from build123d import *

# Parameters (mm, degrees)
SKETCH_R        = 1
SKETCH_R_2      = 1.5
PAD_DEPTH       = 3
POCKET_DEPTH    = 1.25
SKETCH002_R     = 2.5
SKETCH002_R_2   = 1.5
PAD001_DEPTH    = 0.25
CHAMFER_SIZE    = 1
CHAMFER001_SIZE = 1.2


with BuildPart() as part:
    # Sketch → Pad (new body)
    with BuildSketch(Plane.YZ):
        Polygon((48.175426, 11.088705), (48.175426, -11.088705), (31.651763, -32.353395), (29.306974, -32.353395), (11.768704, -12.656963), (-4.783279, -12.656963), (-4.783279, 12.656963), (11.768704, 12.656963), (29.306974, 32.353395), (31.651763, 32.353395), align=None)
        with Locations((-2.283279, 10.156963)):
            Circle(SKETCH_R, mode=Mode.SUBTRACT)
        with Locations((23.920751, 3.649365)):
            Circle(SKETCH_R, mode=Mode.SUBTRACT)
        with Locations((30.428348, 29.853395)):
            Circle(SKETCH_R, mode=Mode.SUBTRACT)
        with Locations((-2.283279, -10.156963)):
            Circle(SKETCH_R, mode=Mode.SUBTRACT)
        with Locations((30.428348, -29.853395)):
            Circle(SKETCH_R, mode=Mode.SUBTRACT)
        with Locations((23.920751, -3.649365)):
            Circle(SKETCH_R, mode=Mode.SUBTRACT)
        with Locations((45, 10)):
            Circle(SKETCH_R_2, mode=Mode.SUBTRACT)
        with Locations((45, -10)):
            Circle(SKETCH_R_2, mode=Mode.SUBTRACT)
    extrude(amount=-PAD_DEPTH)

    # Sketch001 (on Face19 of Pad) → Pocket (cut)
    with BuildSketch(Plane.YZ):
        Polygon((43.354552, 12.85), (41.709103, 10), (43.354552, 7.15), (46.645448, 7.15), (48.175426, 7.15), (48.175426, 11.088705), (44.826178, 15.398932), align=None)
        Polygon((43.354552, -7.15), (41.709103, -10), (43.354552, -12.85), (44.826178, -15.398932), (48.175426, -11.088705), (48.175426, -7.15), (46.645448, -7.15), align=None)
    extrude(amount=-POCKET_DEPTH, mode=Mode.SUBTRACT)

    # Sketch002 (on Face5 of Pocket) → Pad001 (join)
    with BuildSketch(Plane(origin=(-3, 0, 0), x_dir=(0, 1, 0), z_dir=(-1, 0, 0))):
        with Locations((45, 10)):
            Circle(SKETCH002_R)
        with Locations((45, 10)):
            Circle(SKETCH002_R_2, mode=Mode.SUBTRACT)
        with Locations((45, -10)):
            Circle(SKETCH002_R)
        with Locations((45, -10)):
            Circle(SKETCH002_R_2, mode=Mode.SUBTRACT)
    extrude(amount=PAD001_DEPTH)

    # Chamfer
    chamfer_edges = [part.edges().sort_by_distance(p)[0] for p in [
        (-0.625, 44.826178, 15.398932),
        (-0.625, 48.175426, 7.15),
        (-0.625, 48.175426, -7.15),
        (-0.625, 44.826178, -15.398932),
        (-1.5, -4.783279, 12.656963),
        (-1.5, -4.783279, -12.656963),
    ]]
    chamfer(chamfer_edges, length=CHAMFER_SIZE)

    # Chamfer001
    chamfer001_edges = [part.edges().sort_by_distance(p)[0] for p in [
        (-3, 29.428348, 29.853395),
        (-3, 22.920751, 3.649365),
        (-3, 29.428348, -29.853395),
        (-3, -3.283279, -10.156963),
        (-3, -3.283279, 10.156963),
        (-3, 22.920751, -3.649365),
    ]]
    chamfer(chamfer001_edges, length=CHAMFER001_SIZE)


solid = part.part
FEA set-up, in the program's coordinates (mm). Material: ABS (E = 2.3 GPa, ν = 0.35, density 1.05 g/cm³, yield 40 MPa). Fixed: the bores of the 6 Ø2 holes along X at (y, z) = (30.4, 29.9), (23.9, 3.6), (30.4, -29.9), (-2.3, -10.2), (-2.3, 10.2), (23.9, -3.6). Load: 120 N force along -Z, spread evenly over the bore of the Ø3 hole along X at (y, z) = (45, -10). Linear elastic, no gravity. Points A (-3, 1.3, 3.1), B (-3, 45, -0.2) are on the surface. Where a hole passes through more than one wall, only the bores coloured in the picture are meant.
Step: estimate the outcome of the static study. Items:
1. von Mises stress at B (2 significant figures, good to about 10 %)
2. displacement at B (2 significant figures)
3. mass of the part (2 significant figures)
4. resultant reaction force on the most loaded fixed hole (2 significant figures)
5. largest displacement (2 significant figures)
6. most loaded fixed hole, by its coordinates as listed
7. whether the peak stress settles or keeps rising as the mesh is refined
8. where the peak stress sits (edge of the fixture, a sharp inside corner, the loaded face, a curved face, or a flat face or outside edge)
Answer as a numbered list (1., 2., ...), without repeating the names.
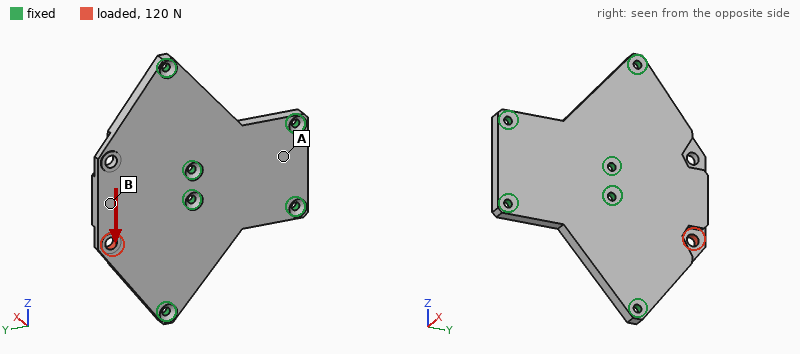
1. 3.6 MPa
2. 41 µm
3. 6.3 g
4. 56 N
5. 61 µm
6. (30.4, -29.9)
7. keeps rising
8. edge of the fixture
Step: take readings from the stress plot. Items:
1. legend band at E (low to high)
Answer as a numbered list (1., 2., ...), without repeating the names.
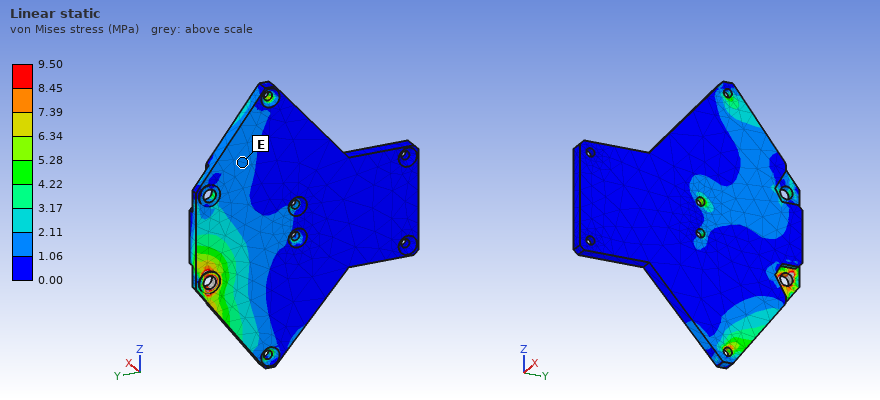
1. 1.06 to 2.11 MPa
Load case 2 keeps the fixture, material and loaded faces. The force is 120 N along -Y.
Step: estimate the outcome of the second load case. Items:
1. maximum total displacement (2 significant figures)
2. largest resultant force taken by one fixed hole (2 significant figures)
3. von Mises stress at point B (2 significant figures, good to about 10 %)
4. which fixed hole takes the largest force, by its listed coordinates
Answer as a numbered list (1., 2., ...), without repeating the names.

1. 0.21 mm
2. 52 N
3. 1.6 MPa
4. (23.9, -3.6)
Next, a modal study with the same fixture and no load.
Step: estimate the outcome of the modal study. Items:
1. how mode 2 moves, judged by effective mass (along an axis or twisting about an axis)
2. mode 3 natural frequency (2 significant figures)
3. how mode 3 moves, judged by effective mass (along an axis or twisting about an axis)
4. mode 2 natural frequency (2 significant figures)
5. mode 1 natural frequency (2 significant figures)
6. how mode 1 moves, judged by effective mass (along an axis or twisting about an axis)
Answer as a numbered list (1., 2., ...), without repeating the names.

1. twisting about Y
2. 4000 Hz
3. along X
4. 2800 Hz
5. 1300 Hz
6. along X
